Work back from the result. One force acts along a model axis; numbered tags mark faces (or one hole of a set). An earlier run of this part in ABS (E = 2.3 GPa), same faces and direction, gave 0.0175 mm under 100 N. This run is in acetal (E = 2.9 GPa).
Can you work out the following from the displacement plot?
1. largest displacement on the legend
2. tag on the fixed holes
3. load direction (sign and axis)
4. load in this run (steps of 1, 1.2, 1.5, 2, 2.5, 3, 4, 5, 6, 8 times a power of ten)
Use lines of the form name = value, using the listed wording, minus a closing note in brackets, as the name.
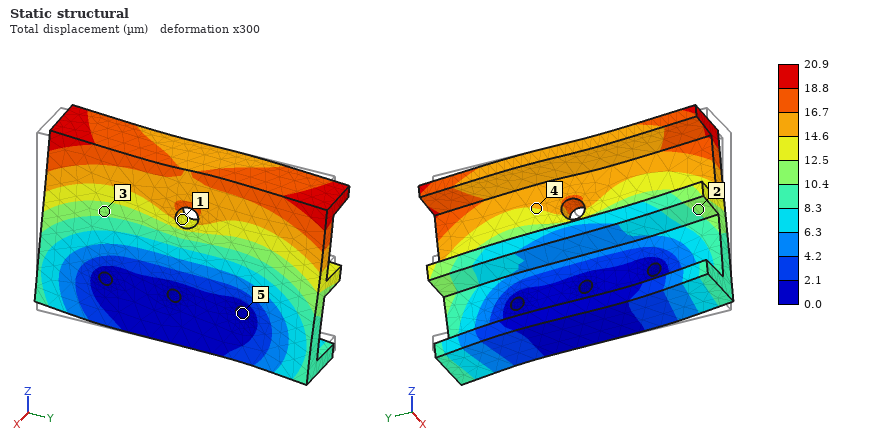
largest displacement on the legend = 20.9 µm
tag on the fixed holes = 5
load direction = +Y
load in this run = 150 N
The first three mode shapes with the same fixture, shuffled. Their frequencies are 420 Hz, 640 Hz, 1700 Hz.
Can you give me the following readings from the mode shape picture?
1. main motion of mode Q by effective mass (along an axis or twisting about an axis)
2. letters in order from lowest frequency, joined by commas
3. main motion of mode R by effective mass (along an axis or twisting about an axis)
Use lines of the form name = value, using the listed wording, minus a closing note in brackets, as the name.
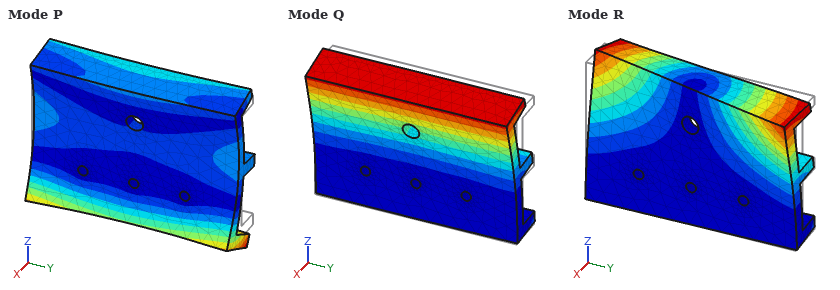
main motion of mode Q by effective mass = along X
letters in order from lowest frequency, joined by commas = Q, R, P
main motion of mode R by effective mass = twisting about Z
